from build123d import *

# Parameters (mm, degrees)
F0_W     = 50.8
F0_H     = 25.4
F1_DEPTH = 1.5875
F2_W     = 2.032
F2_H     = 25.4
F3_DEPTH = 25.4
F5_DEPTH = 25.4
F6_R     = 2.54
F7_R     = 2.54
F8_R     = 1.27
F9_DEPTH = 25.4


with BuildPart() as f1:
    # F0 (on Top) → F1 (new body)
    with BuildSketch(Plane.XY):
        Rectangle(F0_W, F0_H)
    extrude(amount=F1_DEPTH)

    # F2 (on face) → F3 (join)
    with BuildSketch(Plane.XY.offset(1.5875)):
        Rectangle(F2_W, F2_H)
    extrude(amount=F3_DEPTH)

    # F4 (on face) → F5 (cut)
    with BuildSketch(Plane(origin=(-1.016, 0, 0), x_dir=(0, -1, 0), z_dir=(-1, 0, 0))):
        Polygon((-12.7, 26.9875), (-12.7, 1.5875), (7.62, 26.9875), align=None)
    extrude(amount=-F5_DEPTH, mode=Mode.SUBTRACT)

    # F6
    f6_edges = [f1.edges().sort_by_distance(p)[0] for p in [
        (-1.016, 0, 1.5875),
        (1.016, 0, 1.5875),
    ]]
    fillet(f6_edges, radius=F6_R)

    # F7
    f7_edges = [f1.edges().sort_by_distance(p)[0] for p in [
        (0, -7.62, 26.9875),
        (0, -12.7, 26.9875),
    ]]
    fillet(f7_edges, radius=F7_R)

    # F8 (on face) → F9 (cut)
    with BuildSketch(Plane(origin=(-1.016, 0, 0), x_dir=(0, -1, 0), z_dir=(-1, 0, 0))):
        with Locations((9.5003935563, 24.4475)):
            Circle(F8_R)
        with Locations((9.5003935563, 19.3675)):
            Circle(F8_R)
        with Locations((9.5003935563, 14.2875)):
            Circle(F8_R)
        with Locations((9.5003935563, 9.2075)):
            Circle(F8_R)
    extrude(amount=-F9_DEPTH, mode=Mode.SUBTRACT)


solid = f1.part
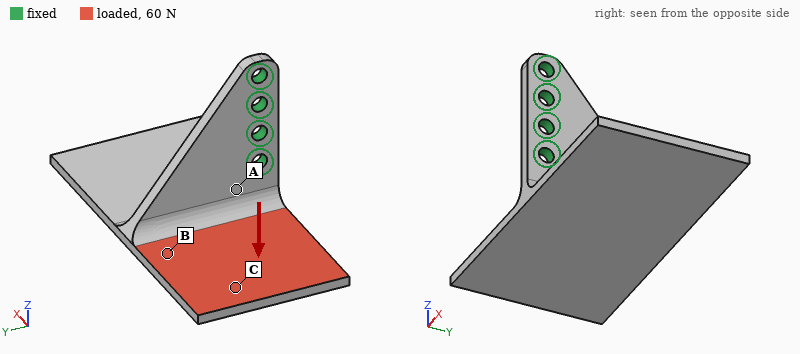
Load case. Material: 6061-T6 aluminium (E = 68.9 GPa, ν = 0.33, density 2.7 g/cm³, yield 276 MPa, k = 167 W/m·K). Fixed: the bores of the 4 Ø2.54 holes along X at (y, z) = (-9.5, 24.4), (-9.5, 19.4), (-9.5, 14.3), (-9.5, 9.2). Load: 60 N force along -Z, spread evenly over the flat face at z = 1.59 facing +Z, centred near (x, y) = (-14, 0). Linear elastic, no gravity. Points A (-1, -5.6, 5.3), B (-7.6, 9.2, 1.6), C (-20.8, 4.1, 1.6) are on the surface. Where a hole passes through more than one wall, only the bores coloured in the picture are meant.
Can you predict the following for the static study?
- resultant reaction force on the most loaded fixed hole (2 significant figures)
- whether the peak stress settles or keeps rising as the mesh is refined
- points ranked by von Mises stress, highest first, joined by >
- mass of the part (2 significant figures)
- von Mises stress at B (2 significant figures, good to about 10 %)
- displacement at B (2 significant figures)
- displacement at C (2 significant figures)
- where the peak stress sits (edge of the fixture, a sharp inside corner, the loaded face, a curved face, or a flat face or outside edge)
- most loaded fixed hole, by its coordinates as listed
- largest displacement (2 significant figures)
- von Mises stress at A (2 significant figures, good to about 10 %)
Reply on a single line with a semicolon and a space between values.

75 N; keeps rising; A > B > C; 7.7 g; 35 MPa; 0.098 mm; 0.29 mm; edge of the fixture; (-9.5, 9.2); 0.38 mm; 65 MPa
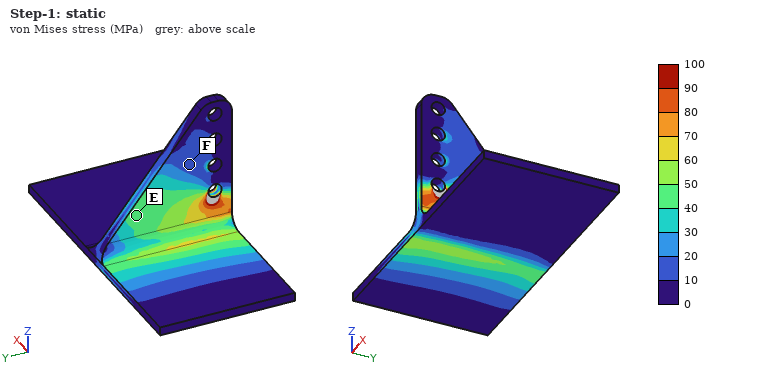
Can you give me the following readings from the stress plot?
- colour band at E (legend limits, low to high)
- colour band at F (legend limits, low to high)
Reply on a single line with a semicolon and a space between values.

40 to 50 MPa; 10 to 20 MPa
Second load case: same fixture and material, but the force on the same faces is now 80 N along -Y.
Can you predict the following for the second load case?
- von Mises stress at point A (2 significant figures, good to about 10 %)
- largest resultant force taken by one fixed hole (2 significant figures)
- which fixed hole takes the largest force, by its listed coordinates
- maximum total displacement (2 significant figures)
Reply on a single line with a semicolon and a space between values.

49 MPa; 120 N; (-9.5, 9.2); 0.24 mm
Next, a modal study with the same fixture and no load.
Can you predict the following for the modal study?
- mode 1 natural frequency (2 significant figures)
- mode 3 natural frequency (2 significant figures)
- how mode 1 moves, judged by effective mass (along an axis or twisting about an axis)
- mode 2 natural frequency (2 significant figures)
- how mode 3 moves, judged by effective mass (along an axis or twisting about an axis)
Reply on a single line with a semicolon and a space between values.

1200 Hz; 2400 Hz; along X; 1700 Hz; along Z
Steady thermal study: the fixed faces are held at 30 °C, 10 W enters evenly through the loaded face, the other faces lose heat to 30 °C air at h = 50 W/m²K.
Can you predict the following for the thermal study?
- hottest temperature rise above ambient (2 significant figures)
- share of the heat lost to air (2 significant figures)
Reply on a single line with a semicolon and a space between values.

32 K; 21 %
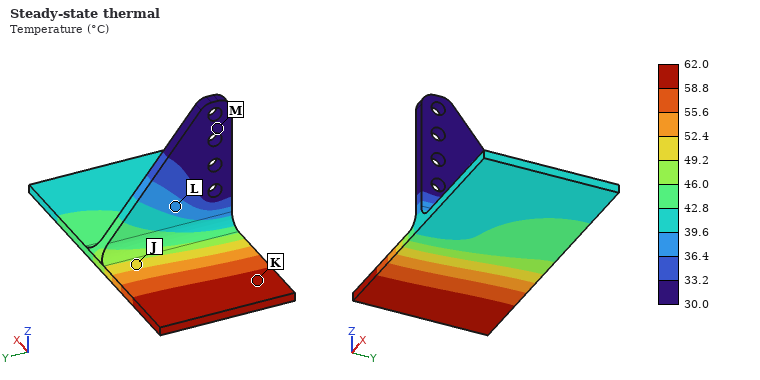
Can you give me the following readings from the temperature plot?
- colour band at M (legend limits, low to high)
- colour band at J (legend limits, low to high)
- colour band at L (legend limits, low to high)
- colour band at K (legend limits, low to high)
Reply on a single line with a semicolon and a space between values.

30.0 to 33.2 °C; 49.2 to 52.4 °C; 36.4 to 39.6 °C; 58.8 to 62.0 °C
